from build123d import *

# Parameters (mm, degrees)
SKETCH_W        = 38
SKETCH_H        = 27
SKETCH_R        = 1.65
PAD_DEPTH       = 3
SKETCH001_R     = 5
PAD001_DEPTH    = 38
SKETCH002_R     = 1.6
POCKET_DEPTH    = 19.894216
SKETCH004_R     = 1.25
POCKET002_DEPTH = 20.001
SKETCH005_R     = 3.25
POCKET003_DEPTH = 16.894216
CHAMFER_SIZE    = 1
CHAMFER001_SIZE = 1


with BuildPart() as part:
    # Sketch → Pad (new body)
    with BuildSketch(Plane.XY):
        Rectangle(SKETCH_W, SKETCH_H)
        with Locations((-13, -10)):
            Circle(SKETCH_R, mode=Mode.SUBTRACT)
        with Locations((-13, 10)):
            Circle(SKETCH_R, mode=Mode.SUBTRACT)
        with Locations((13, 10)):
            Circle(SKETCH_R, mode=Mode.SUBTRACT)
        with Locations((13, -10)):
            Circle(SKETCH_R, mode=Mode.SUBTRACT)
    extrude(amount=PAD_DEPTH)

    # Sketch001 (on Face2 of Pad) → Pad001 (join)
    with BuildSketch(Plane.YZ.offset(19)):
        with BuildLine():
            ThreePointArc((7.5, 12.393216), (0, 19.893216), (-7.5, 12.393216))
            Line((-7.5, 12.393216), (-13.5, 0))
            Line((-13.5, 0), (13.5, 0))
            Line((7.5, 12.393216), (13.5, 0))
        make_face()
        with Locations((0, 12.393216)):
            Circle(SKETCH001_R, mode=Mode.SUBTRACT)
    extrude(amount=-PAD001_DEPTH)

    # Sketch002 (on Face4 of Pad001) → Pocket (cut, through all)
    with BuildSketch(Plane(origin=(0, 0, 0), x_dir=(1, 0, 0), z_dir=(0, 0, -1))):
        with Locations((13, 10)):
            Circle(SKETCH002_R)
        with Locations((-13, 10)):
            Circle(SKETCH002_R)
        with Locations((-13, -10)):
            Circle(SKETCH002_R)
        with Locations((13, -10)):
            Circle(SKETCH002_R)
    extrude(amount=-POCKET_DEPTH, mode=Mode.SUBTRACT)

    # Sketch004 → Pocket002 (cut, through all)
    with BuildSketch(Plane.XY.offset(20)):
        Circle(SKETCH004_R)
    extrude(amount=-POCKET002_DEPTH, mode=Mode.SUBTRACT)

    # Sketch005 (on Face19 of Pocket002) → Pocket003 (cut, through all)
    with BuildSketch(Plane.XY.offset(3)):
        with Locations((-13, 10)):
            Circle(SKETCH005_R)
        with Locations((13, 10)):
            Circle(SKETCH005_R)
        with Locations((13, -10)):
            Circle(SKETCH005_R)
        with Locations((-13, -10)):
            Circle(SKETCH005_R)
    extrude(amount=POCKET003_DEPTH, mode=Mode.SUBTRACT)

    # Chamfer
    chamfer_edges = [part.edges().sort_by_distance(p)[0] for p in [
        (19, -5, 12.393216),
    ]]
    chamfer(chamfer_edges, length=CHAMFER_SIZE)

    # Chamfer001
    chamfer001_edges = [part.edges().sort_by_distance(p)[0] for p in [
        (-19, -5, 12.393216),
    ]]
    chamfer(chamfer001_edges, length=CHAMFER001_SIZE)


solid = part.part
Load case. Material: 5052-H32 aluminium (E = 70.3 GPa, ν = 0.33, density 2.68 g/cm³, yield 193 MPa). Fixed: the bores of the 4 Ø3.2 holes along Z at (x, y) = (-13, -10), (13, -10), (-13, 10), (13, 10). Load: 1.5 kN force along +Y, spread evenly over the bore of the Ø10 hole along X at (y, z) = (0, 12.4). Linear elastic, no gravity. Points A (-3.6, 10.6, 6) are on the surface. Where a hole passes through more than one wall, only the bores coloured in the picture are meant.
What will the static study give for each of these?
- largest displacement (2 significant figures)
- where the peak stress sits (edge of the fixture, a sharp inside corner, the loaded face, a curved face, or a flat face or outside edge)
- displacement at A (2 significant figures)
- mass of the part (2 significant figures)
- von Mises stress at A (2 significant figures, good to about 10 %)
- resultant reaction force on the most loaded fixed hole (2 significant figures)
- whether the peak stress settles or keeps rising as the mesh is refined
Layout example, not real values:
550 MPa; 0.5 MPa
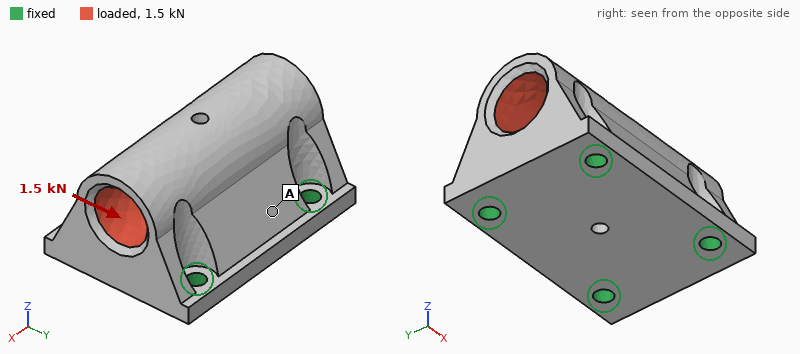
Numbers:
9.9 µm; edge of the fixture; 3.9 µm; 26 g; 6.0 MPa; 580 N; keeps rising
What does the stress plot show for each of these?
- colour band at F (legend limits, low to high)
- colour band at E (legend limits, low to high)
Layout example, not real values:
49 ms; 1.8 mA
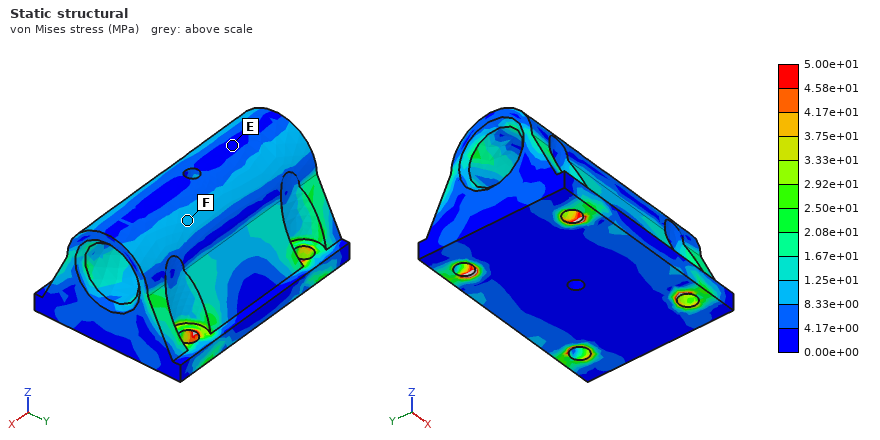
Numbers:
8.33e+00 to 1.25e+01 MPa; 0.00e+00 to 4.17e+00 MPa
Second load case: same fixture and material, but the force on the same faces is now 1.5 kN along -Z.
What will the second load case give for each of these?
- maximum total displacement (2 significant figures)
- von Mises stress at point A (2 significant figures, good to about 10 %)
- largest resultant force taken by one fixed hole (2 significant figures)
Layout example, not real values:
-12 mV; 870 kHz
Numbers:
3.4 µm; 4.4 MPa; 400 N
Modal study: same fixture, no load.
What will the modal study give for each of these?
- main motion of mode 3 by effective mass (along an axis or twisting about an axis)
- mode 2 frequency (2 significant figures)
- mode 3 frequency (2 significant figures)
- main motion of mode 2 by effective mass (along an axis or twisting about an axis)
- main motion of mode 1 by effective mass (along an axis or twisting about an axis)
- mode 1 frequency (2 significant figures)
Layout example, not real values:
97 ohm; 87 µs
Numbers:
along Z; 24 kHz; 26 kHz; along X; along Y; 21 kHz
